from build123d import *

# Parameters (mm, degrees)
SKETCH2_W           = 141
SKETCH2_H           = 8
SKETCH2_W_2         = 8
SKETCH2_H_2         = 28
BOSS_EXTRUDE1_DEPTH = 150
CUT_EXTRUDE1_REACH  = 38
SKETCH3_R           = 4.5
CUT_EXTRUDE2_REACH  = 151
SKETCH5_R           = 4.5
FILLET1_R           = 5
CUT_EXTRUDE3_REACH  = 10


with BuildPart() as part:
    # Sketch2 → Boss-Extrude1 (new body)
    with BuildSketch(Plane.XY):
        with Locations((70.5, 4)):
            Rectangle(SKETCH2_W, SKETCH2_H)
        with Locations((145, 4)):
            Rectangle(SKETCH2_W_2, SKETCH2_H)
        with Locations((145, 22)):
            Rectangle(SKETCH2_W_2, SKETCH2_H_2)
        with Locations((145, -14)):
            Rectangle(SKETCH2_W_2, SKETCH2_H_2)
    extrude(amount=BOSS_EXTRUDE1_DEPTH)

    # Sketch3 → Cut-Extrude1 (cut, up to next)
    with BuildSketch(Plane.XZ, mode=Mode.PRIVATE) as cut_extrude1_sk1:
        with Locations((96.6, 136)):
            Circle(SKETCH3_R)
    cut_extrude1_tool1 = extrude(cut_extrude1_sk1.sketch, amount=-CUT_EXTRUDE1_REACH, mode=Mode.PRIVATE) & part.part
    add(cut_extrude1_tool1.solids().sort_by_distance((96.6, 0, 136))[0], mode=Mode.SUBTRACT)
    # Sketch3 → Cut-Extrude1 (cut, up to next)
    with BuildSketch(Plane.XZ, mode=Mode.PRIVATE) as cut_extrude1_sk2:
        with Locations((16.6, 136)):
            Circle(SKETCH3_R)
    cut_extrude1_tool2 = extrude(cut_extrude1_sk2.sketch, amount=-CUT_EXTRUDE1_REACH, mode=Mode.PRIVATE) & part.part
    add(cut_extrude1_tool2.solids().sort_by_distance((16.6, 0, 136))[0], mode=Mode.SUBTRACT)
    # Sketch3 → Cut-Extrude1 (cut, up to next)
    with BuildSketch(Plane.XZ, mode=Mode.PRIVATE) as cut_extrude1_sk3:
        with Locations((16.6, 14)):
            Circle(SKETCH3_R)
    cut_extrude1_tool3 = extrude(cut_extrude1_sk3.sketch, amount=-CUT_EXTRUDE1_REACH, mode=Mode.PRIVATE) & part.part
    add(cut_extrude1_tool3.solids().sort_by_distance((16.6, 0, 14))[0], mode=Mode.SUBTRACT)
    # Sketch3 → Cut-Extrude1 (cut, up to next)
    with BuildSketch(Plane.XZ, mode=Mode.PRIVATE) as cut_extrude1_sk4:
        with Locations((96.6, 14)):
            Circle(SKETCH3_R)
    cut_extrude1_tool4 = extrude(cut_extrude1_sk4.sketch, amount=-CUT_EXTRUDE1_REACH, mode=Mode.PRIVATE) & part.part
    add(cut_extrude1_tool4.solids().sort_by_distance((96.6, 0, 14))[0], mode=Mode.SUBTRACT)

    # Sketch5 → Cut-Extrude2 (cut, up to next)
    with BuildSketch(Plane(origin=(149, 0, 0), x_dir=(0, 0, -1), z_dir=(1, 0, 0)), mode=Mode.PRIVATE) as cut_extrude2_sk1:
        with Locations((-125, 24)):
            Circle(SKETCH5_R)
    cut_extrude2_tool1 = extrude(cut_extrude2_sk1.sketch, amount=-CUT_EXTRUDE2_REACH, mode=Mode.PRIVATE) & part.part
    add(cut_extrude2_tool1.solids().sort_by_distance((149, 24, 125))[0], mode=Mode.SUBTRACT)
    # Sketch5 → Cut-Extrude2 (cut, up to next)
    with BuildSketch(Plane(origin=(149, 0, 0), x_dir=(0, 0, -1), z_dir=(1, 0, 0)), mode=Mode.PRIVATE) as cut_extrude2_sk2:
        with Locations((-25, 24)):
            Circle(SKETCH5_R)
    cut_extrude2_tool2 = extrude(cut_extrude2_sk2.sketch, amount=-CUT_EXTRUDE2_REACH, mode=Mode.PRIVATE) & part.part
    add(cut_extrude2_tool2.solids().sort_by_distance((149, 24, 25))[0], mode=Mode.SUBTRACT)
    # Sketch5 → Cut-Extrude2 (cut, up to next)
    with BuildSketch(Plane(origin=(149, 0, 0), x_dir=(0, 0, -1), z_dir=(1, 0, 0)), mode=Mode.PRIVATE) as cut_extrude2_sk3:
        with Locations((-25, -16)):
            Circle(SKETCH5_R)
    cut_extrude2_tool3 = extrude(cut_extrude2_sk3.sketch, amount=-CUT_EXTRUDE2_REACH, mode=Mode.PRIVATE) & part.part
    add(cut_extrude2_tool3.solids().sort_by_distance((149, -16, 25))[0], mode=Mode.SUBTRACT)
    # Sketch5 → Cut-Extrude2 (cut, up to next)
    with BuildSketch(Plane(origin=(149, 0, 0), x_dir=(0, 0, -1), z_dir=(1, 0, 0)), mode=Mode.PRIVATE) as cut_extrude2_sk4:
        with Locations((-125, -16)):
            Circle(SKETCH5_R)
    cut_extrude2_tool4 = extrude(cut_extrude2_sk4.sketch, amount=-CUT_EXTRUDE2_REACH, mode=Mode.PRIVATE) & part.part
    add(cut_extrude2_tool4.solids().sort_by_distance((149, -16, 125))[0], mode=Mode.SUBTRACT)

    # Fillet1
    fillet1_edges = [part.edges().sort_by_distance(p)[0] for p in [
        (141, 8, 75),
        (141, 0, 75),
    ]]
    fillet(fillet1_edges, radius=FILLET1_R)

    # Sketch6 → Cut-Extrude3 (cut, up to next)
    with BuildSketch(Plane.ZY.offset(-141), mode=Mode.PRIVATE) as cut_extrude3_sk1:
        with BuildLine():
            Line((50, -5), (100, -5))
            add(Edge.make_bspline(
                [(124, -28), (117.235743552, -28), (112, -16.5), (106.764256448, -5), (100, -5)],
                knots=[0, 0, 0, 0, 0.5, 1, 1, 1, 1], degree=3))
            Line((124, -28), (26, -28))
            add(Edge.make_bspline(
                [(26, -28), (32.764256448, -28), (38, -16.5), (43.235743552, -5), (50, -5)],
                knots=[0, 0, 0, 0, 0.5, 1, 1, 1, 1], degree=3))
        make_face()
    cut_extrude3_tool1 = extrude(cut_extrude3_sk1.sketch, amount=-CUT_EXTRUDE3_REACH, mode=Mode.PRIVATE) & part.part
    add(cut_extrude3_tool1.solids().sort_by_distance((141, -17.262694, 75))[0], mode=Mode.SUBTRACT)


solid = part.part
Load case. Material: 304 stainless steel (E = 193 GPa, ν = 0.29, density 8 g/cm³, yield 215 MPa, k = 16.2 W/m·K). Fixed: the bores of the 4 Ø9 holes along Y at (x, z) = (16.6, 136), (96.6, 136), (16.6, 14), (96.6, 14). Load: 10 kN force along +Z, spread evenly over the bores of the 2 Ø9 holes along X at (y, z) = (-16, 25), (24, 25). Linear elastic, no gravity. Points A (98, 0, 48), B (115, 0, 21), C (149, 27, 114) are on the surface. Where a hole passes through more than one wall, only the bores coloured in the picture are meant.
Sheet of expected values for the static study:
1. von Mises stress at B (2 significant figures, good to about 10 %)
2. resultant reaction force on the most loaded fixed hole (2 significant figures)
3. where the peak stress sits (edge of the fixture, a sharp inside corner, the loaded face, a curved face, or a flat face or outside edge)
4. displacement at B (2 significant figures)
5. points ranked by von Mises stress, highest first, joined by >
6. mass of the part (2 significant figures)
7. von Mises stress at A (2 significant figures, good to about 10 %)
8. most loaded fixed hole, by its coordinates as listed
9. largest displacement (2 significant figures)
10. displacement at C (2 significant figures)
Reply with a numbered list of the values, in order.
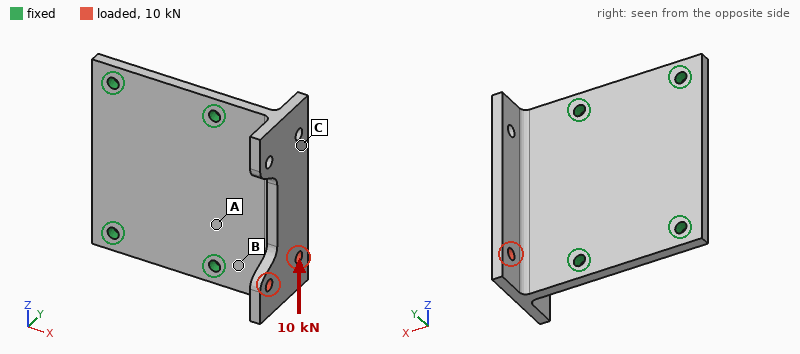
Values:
1. 26 MPa
2. 6.4 kN
3. a sharp inside corner
4. 4.7 µm
5. B > A > C
6. 1.8 kg
7. 11 MPa
8. (96.6, 14)
9. 27 µm
10. 9.2 µm
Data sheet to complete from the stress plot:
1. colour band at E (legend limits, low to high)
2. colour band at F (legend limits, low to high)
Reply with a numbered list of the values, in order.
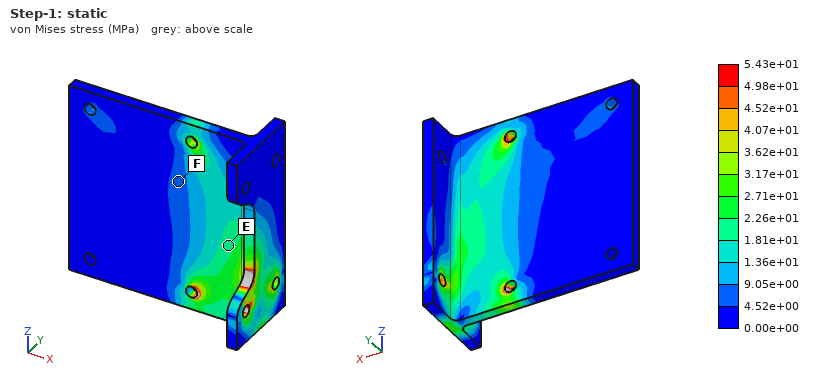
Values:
1. 1.81e+01 to 2.26e+01 MPa
2. 4.52e+00 to 9.05e+00 MPa
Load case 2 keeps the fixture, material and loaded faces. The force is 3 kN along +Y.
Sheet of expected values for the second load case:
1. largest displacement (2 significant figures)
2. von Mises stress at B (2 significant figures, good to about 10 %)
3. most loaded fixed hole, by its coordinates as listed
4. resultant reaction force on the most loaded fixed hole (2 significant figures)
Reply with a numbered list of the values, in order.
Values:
1. 0.25 mm
2. 93 MPa
3. (96.6, 14)
4. 3.1 kN
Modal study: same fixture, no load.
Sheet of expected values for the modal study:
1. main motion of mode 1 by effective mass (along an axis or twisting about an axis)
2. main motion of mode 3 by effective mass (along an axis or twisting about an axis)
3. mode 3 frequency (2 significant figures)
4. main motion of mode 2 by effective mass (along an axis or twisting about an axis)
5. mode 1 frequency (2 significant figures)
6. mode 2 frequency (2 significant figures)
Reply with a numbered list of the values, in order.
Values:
1. along Y
2. along Y
3. 2500 Hz
4. twisting about X
5. 940 Hz
6. 1600 Hz
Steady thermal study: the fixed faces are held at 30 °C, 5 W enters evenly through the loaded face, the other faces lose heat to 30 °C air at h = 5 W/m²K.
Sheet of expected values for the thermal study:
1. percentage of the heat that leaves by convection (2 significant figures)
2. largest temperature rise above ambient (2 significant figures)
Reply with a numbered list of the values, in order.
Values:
1. 35 %
2. 30 K
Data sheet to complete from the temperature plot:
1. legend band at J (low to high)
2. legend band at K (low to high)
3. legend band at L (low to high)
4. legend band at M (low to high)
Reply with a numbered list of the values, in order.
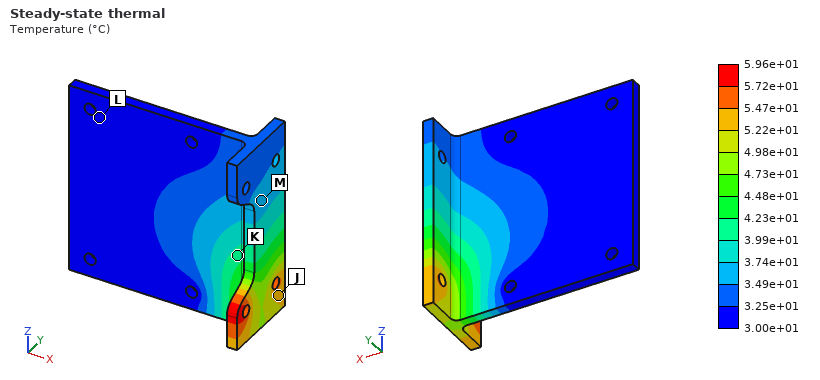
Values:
1. 5.22e+01 to 5.47e+01 °C
2. 3.99e+01 to 4.23e+01 °C
3. 3.00e+01 to 3.25e+01 °C
4. 3.49e+01 to 3.74e+01 °C
